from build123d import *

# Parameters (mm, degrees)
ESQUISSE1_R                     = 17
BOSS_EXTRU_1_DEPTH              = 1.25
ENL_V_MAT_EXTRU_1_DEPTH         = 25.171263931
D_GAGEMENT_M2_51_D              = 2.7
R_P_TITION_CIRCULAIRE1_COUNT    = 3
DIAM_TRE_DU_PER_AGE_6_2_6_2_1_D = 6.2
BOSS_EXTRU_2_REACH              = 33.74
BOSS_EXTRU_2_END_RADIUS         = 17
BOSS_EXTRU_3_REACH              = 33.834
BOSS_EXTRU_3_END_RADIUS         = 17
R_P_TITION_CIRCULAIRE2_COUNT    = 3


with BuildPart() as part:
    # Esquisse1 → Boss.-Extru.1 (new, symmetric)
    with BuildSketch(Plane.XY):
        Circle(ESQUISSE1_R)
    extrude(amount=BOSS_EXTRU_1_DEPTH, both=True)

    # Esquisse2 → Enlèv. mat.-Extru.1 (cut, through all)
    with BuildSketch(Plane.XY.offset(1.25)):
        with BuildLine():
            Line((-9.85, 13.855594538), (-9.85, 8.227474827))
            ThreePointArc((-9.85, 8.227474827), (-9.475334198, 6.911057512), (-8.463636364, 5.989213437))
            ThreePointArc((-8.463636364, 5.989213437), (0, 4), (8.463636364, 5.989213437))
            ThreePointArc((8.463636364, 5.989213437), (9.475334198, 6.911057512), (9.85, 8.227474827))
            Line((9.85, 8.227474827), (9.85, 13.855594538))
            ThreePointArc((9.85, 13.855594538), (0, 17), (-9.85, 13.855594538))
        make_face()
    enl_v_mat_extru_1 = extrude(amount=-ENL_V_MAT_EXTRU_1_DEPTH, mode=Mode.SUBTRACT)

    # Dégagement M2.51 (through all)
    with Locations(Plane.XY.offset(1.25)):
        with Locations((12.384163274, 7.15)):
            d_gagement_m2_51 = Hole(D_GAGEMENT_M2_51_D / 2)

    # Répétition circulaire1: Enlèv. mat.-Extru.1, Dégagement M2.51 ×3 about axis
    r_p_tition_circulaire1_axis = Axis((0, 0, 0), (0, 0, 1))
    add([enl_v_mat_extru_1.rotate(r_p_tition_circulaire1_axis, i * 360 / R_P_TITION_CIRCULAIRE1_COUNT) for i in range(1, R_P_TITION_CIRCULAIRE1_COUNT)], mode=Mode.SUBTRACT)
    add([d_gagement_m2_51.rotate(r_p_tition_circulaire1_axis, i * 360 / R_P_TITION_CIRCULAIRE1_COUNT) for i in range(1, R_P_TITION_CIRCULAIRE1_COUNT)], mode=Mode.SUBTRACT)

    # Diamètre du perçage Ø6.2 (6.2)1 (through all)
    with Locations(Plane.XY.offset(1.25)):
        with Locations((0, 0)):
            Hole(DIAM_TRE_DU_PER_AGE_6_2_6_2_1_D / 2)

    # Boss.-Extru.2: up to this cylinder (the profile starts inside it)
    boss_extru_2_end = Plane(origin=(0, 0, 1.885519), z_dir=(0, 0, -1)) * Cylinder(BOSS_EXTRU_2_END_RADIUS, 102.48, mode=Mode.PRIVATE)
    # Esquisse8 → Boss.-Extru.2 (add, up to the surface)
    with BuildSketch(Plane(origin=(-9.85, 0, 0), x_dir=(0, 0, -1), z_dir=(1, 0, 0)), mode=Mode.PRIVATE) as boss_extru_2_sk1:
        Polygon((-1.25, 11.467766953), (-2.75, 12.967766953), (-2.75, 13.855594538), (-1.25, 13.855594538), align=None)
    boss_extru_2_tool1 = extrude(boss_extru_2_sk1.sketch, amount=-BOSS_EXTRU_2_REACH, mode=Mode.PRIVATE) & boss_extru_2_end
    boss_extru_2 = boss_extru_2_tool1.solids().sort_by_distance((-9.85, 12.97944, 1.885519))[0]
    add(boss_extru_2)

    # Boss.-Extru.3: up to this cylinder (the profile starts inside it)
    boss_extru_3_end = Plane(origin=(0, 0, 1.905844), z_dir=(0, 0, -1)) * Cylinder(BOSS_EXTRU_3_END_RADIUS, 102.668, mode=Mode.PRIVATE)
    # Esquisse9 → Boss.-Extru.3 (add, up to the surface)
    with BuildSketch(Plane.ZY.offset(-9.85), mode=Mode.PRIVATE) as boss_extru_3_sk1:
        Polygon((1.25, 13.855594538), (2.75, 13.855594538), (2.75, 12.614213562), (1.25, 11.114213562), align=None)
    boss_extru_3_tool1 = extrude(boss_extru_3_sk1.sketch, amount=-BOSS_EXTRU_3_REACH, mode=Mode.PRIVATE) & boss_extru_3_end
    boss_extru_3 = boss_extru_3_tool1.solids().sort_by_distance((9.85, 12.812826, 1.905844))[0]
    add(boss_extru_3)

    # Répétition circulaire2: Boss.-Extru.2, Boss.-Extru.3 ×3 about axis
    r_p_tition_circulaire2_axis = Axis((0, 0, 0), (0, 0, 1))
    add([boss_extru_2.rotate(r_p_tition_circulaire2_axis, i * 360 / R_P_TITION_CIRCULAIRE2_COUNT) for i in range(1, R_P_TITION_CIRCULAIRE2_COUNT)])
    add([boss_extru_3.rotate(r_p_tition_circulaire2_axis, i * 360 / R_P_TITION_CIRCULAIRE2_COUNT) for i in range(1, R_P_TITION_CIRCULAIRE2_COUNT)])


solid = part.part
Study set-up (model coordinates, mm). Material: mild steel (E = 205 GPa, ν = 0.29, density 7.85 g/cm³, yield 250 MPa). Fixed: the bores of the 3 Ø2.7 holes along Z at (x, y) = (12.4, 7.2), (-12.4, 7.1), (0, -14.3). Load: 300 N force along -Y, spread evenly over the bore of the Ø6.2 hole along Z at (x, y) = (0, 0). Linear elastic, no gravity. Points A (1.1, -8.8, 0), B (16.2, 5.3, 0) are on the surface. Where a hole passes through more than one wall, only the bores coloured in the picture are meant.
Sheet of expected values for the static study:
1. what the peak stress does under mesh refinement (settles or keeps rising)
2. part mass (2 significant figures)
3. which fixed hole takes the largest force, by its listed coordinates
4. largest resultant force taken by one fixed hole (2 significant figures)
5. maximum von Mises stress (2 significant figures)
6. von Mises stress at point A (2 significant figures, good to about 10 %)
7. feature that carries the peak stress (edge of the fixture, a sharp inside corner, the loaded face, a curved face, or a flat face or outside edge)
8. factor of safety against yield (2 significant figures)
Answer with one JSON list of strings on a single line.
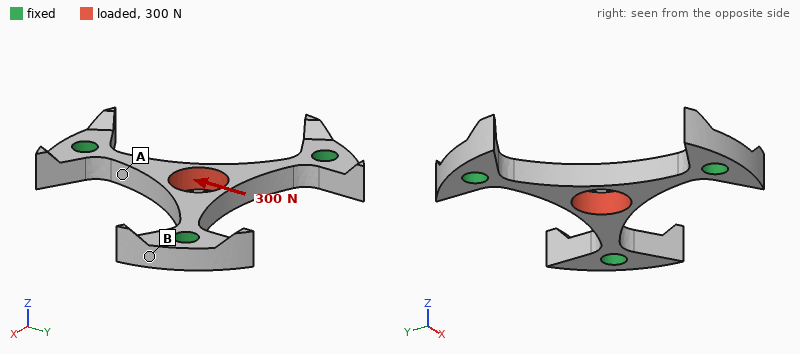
["settles", "4.2 g", "(0, -14.3)", "200 N", "130 MPa", "37 MPa", "the loaded face", "2.0"]
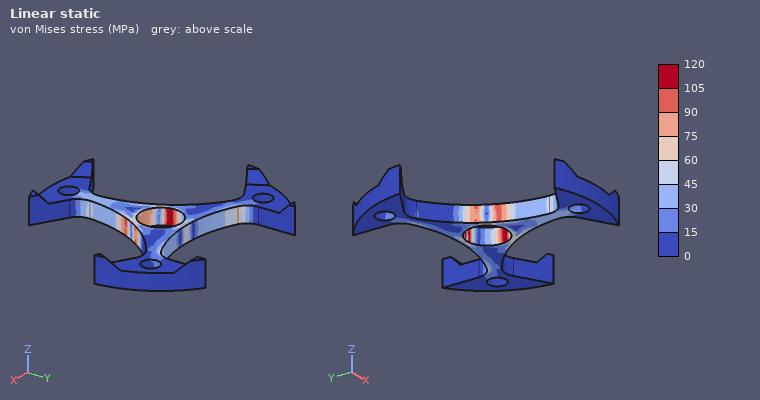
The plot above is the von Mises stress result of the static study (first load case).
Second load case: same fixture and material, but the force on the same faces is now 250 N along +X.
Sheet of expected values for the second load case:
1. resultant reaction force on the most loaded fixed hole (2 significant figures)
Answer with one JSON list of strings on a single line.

["150 N"]
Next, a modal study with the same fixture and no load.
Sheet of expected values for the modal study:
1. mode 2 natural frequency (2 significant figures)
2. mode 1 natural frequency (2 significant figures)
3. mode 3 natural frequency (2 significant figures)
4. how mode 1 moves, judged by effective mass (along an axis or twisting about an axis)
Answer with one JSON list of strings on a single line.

["36 kHz", "18 kHz", "37 kHz", "along Z"]
